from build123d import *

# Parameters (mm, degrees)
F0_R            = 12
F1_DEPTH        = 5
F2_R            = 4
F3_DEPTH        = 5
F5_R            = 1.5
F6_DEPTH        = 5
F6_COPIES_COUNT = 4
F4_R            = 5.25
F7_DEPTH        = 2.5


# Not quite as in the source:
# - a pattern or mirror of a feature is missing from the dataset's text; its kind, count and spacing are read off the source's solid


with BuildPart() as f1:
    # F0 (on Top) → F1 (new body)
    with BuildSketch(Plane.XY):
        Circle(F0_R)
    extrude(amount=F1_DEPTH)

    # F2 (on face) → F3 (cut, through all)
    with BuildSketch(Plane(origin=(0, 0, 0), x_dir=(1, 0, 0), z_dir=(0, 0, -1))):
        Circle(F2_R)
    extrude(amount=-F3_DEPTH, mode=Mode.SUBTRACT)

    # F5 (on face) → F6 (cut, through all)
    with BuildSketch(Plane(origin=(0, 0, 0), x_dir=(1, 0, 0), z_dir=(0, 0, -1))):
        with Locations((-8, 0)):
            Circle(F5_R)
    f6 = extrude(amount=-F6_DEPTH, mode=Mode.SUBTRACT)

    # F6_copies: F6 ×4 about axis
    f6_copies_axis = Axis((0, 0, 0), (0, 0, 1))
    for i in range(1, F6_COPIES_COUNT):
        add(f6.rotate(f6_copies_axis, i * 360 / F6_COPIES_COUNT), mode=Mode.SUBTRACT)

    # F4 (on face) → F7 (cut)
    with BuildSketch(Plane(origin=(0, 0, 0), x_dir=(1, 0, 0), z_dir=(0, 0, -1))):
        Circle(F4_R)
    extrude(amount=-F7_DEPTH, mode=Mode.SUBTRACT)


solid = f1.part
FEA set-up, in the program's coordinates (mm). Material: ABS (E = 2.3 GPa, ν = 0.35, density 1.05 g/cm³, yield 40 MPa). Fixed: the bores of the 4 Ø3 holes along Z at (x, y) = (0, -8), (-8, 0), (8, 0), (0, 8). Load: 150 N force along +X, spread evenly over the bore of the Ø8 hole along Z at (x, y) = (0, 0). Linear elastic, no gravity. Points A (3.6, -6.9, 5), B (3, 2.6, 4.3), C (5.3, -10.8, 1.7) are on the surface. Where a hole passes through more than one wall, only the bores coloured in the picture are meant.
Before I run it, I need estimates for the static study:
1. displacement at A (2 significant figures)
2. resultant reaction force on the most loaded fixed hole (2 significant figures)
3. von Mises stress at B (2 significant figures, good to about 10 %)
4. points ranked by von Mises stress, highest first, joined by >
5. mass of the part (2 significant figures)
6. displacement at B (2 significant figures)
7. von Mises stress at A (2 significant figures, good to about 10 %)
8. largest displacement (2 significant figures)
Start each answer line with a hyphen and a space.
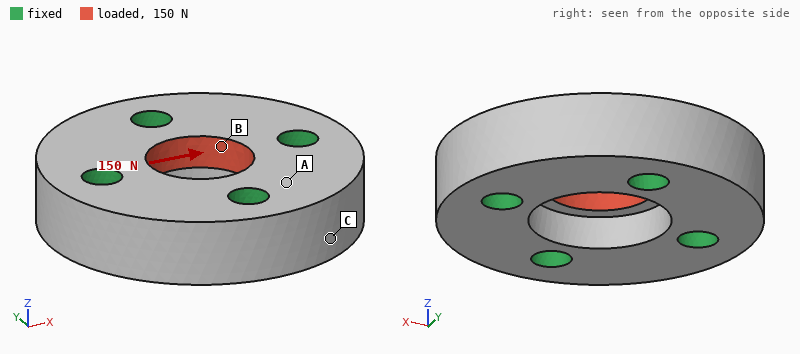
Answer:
- 1.9 µm
- 43 N
- 3.1 MPa
- B > A > C
- 1.9 g
- 5.4 µm
- 1.0 MPa
- 6.0 µm
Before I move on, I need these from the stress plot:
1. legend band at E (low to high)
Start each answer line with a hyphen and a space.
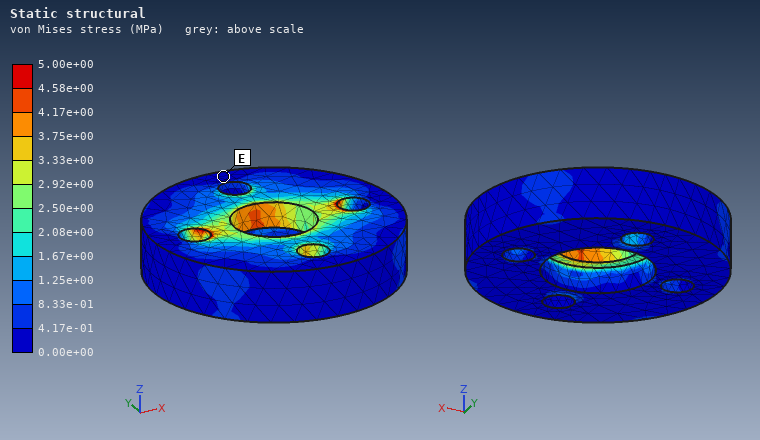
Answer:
- 0.00e+00 to 4.17e-01 MPa
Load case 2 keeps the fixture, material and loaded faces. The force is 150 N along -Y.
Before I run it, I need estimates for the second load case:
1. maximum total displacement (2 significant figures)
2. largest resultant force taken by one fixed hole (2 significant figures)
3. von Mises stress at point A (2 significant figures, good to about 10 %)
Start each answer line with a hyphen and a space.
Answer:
- 6.0 µm
- 43 N
- 1.2 MPa
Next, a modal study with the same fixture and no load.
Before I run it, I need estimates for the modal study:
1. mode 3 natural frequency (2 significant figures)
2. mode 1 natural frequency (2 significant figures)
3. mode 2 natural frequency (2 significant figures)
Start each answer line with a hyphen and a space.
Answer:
- 24 kHz
- 24 kHz
- 24 kHz
